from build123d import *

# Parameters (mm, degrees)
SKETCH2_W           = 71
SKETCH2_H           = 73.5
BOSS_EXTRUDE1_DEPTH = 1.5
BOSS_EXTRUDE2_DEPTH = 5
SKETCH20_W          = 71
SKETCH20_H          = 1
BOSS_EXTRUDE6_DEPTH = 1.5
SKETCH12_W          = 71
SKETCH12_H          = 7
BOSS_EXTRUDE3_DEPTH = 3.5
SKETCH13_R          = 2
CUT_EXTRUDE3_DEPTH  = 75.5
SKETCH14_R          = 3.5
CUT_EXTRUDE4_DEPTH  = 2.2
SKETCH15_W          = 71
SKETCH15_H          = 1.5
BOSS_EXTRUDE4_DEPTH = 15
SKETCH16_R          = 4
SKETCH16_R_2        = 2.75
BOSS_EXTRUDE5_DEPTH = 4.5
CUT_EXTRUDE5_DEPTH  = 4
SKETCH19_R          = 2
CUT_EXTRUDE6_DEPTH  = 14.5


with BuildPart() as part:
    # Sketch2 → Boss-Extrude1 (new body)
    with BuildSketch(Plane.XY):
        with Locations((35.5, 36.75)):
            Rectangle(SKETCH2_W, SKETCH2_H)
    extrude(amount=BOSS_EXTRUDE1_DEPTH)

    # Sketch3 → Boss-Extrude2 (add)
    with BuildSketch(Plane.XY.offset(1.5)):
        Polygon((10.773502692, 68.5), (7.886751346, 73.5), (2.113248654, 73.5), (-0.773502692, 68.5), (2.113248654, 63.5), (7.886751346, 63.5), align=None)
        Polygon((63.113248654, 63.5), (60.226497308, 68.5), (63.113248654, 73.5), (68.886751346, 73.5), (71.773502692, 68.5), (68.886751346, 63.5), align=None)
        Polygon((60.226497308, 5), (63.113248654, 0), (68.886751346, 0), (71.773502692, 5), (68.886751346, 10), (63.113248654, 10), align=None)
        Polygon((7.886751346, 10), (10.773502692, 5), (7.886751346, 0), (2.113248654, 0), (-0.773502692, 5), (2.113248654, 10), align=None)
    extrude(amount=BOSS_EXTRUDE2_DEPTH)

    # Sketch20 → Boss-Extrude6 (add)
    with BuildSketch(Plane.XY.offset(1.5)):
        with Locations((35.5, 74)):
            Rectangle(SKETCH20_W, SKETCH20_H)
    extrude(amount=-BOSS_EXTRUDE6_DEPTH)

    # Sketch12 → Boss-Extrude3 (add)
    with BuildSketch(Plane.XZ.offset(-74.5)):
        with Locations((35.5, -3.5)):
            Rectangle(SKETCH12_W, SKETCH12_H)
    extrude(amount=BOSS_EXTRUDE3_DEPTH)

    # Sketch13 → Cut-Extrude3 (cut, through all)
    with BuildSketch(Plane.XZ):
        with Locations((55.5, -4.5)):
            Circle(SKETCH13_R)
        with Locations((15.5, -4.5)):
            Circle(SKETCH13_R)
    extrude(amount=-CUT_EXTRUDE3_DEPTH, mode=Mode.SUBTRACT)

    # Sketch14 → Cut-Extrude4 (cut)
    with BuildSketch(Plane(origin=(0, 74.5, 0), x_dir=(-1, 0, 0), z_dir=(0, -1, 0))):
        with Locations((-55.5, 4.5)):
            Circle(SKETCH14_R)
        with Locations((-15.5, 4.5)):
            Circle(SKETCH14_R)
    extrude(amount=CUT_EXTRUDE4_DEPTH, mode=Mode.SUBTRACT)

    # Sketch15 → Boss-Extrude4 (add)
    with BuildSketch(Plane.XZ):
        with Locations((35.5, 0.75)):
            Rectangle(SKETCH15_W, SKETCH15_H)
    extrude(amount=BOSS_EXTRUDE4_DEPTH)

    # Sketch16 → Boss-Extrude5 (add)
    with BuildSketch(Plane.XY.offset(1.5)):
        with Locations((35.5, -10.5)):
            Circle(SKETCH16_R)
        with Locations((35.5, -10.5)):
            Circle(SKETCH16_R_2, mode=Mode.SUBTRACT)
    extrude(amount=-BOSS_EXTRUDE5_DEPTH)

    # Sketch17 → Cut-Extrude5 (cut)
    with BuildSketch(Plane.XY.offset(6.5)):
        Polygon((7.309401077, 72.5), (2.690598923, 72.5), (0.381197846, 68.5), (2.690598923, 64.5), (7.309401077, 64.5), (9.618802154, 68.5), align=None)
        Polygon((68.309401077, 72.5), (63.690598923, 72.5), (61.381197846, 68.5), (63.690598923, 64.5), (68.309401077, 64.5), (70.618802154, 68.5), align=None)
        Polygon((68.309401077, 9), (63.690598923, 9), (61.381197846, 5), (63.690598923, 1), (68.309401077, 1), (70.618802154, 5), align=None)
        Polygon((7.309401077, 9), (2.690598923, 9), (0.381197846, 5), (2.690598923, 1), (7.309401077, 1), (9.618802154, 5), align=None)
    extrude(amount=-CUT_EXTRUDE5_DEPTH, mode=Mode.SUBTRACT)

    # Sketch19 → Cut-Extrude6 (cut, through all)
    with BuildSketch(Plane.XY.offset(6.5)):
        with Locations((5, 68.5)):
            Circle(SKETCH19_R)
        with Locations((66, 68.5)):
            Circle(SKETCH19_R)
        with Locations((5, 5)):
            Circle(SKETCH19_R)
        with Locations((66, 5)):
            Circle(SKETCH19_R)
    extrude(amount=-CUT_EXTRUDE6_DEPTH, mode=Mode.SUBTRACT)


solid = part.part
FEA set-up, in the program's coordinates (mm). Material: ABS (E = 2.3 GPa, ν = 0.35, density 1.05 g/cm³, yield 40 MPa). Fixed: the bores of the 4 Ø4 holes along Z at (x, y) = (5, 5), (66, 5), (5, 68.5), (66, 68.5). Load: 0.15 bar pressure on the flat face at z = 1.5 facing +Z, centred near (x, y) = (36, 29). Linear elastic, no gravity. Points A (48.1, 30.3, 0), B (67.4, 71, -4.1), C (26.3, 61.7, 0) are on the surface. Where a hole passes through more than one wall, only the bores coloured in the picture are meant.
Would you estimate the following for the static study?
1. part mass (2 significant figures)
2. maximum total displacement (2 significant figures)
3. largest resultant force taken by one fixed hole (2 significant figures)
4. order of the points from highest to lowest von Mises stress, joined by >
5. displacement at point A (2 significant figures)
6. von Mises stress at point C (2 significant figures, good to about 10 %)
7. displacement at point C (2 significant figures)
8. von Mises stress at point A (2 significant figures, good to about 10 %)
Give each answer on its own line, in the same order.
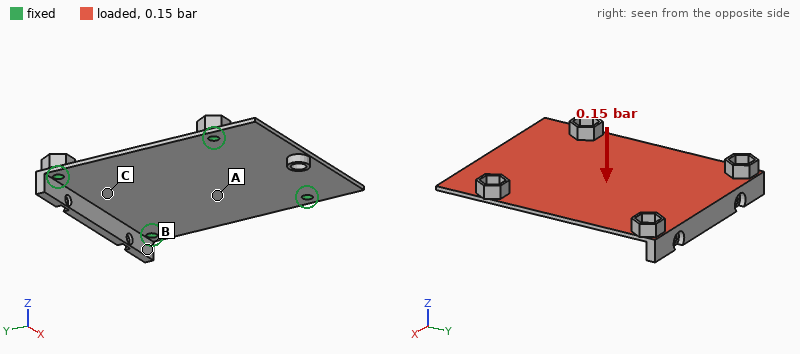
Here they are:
12 g
1.4 mm
29 N
A > C > B
1.2 mm
3.0 MPa
0.42 mm
5.7 MPa
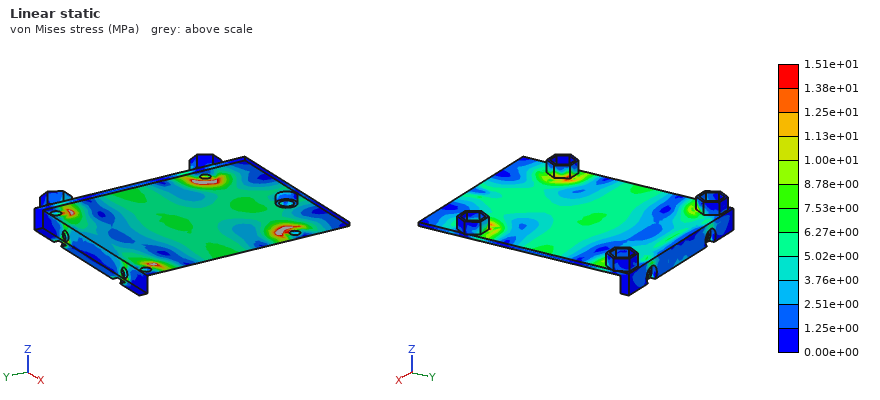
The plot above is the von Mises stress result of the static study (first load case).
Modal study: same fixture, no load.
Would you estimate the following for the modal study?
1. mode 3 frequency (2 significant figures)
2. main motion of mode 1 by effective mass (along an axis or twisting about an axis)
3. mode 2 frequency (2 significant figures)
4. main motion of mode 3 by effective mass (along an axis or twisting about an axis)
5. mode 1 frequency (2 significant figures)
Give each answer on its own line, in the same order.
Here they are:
780 Hz
along Z
590 Hz
twisting about Y
510 Hz
